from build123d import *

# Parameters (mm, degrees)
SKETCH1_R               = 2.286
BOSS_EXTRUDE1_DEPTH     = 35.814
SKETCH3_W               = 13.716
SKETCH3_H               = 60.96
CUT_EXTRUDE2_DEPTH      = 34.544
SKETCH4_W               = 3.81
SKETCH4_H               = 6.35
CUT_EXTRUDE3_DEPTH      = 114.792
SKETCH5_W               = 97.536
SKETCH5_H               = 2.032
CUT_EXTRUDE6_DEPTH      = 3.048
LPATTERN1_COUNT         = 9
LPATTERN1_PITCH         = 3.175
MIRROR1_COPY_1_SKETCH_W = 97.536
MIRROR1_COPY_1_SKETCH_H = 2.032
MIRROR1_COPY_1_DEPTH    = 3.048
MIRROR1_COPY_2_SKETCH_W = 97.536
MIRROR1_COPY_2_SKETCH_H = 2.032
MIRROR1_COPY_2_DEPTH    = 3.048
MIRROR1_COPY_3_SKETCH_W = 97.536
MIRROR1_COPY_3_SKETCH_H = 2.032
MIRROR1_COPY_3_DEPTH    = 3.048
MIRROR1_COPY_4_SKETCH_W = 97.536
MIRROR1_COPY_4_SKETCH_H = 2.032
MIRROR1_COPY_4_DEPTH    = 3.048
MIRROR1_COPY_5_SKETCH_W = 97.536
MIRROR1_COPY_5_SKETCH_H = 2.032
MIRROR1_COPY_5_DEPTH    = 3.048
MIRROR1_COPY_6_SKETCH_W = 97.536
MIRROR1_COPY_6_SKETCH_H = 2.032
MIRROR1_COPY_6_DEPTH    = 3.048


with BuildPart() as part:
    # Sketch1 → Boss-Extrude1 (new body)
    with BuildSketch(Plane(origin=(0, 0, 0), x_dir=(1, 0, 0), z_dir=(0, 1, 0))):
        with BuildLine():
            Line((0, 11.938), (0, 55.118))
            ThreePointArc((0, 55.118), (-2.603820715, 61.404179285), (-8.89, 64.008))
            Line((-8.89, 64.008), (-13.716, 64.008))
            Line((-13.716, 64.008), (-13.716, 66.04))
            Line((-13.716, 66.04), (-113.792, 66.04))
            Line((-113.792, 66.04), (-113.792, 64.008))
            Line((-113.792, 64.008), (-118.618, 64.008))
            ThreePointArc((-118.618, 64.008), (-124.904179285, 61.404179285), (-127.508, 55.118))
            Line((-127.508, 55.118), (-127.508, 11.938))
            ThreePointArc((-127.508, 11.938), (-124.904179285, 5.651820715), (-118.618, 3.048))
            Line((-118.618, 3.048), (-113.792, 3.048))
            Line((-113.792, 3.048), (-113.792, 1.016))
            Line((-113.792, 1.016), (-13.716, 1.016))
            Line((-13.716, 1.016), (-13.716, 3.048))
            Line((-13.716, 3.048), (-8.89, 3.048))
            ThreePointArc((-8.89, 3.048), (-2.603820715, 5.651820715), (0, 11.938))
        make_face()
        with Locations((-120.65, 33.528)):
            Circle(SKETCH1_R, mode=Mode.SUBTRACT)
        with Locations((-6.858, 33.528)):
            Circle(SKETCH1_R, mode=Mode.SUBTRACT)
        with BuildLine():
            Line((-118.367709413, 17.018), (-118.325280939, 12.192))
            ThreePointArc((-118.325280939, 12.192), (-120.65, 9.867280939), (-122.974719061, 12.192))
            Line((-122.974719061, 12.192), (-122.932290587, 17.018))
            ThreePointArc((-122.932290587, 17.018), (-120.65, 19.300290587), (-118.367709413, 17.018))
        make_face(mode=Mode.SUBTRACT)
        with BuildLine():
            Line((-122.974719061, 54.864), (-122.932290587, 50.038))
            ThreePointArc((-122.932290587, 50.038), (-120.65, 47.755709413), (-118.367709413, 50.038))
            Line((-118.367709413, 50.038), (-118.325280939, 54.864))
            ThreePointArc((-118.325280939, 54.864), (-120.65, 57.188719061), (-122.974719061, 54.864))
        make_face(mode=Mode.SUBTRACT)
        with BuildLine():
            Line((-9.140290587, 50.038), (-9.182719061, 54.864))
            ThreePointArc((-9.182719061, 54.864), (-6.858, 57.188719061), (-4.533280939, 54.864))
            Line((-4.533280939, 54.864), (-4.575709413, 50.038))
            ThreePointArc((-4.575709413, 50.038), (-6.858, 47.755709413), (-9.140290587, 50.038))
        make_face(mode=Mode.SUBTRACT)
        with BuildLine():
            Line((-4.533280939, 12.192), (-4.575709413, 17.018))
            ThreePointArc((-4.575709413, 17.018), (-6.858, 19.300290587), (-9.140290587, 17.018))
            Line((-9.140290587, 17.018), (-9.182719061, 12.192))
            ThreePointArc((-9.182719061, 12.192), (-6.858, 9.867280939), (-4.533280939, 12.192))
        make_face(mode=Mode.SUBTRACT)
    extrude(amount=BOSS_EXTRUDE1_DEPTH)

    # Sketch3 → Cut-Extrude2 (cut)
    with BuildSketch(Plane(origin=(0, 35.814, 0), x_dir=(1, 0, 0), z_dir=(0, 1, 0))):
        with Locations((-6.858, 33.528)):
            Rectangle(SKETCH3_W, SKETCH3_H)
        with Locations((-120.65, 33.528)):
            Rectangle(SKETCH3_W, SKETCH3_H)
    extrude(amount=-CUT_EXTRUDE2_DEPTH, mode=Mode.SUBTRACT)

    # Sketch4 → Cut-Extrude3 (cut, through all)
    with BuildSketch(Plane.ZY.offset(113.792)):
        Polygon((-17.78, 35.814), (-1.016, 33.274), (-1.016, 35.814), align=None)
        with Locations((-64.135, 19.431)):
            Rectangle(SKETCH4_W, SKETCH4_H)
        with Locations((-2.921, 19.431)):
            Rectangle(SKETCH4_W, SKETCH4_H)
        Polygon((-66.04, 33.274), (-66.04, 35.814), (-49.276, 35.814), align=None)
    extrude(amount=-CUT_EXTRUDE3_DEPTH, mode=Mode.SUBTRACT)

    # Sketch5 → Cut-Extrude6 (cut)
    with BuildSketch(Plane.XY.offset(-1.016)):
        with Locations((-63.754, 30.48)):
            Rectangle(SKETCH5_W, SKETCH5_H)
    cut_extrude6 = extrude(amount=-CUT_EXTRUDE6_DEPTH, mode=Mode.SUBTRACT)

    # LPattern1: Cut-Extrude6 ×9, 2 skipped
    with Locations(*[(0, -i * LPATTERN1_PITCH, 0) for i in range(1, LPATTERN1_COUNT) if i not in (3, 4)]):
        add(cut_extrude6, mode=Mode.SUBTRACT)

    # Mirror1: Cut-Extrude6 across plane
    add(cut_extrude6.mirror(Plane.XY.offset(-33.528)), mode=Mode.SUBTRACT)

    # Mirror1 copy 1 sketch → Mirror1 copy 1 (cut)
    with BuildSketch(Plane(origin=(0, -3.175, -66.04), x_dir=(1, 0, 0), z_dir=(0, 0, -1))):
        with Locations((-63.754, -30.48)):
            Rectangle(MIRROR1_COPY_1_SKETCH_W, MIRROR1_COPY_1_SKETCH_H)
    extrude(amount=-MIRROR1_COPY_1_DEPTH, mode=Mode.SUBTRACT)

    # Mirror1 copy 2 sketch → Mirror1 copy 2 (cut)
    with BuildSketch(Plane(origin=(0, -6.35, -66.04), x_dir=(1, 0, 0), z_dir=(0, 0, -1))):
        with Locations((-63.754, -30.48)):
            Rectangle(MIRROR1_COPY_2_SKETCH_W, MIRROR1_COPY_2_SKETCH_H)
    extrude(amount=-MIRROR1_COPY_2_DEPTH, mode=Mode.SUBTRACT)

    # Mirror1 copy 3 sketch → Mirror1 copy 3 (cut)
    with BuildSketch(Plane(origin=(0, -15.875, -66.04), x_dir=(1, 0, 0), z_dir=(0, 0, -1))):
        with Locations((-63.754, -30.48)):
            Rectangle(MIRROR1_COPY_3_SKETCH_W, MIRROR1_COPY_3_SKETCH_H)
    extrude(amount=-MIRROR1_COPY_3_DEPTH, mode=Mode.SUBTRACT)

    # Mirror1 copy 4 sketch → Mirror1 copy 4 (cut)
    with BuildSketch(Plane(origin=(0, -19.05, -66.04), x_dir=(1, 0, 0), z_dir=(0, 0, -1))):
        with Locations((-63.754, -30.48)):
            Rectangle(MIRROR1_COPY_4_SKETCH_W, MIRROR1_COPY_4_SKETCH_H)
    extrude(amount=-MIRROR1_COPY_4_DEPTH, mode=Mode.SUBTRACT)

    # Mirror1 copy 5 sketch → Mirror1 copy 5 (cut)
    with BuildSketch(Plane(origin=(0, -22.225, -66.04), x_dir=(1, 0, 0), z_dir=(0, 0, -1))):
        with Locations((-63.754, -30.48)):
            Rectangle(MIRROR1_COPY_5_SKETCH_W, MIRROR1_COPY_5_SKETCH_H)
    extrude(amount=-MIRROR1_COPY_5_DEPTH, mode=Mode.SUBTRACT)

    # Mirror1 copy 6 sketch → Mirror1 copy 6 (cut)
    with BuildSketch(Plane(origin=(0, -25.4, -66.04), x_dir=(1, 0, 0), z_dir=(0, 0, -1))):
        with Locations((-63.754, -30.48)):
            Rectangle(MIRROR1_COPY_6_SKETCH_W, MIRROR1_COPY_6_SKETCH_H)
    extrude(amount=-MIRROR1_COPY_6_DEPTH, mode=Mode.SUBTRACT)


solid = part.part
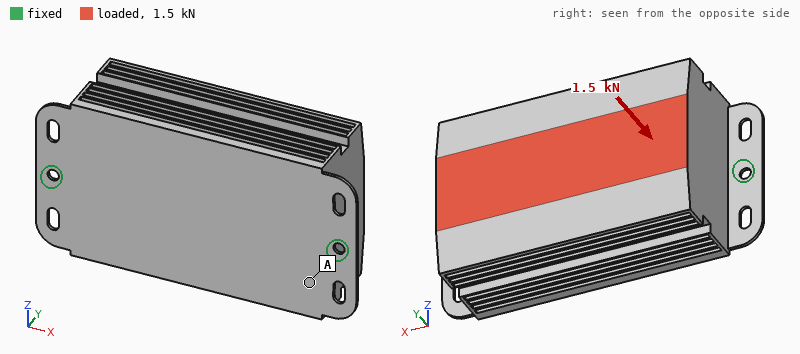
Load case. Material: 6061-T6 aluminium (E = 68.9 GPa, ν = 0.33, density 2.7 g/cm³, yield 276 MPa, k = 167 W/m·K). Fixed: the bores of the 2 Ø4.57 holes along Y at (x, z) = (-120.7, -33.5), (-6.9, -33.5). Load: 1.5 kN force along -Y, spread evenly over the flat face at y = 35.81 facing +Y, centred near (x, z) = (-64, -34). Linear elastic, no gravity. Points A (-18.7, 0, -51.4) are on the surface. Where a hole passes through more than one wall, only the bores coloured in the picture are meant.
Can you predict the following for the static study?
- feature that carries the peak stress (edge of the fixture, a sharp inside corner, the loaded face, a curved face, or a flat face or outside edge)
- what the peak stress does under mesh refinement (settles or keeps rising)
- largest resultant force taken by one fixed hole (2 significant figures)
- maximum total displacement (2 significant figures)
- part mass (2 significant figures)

edge of the fixture
keeps rising
860 N
92 µm
590 g
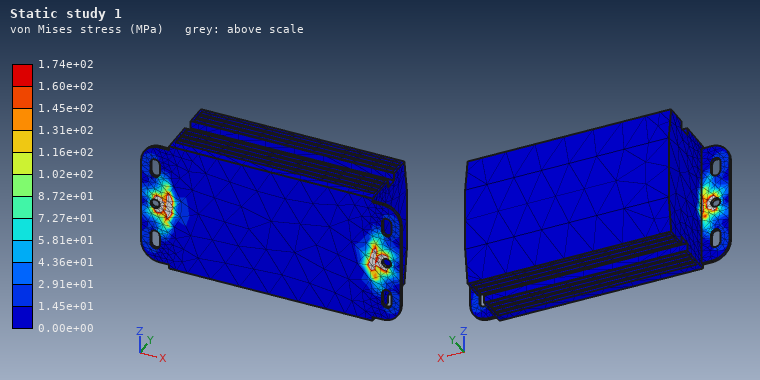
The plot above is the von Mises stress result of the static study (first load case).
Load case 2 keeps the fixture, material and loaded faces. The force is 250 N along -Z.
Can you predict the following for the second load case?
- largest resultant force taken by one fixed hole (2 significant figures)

130 N
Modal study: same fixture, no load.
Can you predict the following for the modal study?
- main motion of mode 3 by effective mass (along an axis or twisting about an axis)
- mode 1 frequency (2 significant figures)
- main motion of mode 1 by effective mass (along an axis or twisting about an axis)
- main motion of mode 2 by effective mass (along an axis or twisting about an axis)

along X
140 Hz
along Z
along Y
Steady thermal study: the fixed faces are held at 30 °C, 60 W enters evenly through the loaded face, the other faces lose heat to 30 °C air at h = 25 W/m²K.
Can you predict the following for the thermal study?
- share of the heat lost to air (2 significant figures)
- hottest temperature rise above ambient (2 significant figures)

44 %
34 K
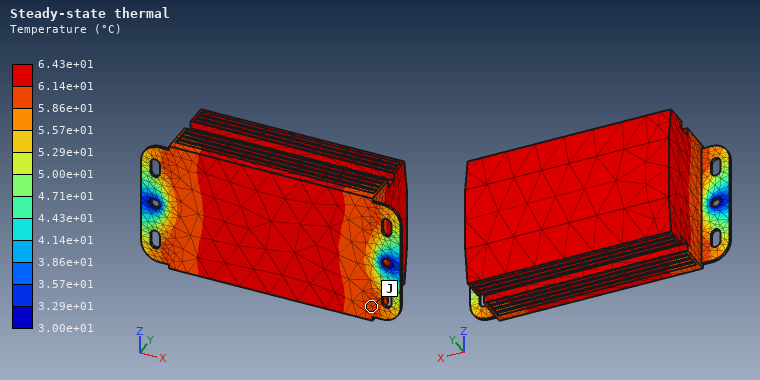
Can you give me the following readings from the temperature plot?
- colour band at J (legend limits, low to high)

5.86e+01 to 6.14e+01 °C
